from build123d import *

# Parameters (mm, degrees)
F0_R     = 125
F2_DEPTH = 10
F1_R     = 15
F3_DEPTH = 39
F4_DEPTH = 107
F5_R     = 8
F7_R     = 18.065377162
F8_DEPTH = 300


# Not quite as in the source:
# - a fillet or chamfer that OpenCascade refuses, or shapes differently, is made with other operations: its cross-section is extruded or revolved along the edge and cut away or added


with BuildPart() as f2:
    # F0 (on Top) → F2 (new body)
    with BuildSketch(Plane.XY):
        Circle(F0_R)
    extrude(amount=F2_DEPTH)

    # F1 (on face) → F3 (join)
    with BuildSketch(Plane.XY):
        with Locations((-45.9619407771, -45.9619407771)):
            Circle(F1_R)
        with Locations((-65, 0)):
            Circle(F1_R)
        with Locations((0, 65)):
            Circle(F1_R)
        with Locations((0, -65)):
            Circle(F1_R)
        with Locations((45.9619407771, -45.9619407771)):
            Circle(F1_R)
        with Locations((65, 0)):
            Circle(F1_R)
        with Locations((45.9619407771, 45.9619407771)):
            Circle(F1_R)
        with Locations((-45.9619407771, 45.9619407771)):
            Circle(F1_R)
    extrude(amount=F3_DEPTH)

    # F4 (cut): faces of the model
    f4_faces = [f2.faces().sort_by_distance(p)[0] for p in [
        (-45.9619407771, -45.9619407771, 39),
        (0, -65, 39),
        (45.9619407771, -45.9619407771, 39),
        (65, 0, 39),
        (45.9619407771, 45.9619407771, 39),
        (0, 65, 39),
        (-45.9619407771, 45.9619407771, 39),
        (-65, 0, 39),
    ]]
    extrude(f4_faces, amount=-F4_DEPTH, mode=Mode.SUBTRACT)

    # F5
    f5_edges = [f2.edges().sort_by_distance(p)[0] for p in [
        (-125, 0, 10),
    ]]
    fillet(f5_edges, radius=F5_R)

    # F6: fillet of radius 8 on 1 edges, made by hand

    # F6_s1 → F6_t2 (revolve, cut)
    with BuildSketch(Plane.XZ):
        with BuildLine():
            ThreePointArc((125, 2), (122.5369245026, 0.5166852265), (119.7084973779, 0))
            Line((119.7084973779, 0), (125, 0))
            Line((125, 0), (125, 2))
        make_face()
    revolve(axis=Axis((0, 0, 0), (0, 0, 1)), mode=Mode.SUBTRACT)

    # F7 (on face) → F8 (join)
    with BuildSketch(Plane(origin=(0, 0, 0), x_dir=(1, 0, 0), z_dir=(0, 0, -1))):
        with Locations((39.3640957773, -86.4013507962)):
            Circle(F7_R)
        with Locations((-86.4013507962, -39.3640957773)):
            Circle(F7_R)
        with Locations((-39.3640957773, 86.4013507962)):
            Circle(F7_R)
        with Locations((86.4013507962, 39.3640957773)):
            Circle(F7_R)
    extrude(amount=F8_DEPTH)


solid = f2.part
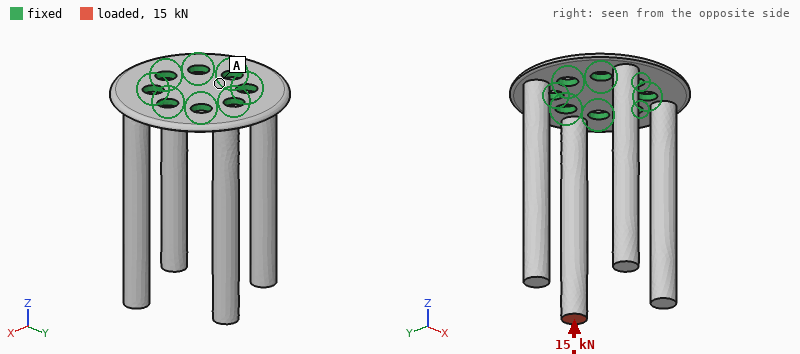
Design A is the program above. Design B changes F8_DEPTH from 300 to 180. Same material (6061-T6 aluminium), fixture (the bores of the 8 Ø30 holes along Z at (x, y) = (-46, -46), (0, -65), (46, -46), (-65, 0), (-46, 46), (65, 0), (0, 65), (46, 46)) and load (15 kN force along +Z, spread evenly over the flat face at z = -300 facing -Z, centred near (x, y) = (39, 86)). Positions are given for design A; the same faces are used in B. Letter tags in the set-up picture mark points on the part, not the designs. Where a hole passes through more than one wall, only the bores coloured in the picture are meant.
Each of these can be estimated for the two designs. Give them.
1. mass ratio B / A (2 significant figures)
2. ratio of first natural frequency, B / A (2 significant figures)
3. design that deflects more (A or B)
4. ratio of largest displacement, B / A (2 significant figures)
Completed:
0.70
2.3
A
0.62
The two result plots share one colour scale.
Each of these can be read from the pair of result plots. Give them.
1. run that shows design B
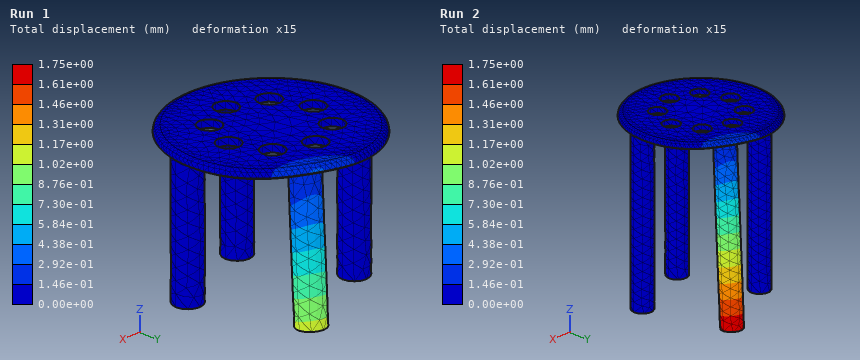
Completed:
Run 1
